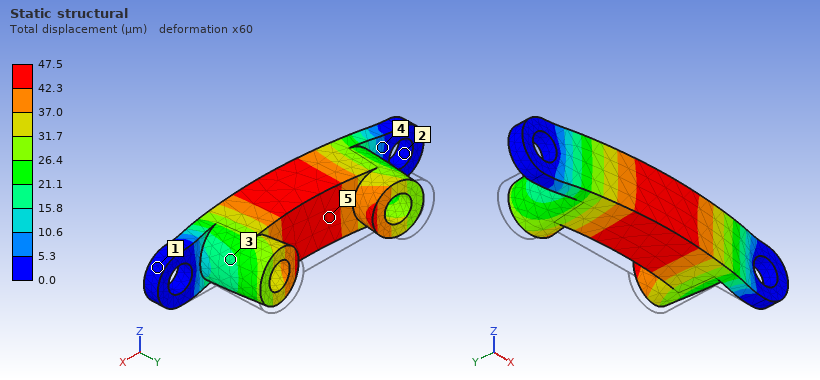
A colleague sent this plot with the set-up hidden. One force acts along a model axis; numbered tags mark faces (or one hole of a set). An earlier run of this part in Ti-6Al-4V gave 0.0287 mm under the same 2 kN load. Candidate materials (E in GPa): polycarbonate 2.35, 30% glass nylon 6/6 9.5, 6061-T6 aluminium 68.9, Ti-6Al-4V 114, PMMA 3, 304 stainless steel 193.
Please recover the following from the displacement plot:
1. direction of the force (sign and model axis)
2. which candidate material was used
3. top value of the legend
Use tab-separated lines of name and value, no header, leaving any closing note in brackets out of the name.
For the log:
direction of the force	-Y
which candidate material was used	6061-T6 aluminium
top value of the legend	47.5 µm
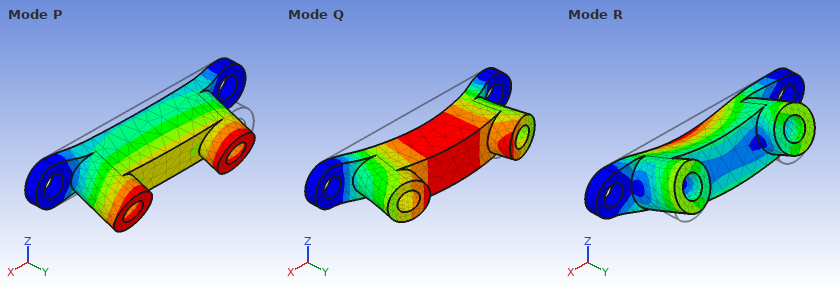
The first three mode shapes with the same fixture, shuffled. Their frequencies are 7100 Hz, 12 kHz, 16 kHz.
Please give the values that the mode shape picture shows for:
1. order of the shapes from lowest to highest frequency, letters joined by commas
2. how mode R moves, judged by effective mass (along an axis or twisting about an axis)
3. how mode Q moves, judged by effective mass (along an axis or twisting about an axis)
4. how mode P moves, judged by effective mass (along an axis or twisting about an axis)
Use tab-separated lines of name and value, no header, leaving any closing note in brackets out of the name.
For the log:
order of the shapes from lowest to highest frequency, letters joined by commas	P, Q, R
how mode R moves, judged by effective mass	along Z
how mode Q moves, judged by effective mass	along Y
how mode P moves, judged by effective mass	along Z
